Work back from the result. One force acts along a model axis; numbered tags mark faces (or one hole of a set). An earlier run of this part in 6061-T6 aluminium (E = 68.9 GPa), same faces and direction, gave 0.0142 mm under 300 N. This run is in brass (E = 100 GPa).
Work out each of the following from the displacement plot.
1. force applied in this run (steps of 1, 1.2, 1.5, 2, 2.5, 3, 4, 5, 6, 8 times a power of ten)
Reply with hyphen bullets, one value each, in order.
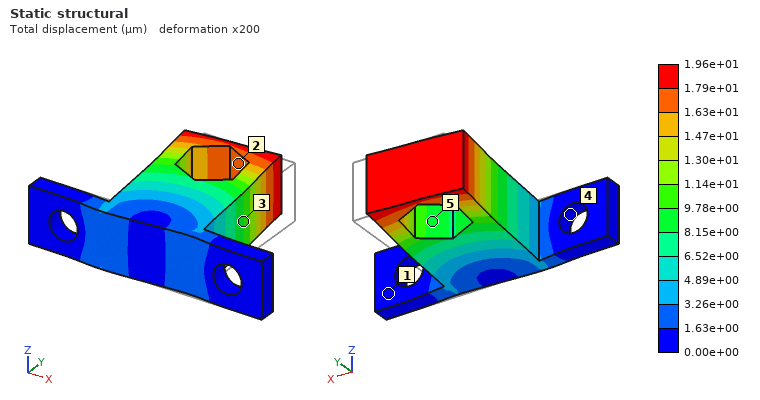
- 600 N
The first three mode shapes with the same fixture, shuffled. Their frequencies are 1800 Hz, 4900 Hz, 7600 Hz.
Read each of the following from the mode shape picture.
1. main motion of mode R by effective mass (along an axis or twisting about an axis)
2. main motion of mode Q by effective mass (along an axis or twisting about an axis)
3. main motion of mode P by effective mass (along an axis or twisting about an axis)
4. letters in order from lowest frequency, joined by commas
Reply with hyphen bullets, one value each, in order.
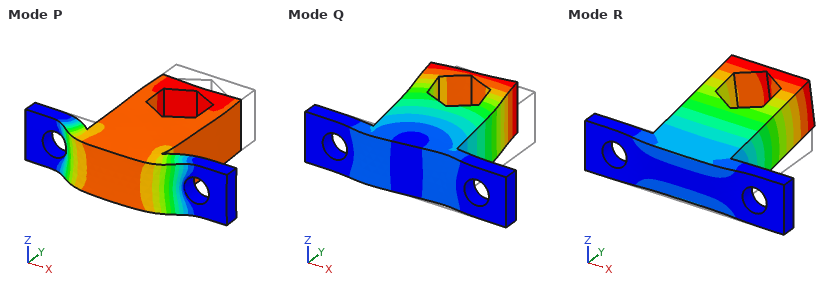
- along Z
- along X
- along Y
- R, Q, P
